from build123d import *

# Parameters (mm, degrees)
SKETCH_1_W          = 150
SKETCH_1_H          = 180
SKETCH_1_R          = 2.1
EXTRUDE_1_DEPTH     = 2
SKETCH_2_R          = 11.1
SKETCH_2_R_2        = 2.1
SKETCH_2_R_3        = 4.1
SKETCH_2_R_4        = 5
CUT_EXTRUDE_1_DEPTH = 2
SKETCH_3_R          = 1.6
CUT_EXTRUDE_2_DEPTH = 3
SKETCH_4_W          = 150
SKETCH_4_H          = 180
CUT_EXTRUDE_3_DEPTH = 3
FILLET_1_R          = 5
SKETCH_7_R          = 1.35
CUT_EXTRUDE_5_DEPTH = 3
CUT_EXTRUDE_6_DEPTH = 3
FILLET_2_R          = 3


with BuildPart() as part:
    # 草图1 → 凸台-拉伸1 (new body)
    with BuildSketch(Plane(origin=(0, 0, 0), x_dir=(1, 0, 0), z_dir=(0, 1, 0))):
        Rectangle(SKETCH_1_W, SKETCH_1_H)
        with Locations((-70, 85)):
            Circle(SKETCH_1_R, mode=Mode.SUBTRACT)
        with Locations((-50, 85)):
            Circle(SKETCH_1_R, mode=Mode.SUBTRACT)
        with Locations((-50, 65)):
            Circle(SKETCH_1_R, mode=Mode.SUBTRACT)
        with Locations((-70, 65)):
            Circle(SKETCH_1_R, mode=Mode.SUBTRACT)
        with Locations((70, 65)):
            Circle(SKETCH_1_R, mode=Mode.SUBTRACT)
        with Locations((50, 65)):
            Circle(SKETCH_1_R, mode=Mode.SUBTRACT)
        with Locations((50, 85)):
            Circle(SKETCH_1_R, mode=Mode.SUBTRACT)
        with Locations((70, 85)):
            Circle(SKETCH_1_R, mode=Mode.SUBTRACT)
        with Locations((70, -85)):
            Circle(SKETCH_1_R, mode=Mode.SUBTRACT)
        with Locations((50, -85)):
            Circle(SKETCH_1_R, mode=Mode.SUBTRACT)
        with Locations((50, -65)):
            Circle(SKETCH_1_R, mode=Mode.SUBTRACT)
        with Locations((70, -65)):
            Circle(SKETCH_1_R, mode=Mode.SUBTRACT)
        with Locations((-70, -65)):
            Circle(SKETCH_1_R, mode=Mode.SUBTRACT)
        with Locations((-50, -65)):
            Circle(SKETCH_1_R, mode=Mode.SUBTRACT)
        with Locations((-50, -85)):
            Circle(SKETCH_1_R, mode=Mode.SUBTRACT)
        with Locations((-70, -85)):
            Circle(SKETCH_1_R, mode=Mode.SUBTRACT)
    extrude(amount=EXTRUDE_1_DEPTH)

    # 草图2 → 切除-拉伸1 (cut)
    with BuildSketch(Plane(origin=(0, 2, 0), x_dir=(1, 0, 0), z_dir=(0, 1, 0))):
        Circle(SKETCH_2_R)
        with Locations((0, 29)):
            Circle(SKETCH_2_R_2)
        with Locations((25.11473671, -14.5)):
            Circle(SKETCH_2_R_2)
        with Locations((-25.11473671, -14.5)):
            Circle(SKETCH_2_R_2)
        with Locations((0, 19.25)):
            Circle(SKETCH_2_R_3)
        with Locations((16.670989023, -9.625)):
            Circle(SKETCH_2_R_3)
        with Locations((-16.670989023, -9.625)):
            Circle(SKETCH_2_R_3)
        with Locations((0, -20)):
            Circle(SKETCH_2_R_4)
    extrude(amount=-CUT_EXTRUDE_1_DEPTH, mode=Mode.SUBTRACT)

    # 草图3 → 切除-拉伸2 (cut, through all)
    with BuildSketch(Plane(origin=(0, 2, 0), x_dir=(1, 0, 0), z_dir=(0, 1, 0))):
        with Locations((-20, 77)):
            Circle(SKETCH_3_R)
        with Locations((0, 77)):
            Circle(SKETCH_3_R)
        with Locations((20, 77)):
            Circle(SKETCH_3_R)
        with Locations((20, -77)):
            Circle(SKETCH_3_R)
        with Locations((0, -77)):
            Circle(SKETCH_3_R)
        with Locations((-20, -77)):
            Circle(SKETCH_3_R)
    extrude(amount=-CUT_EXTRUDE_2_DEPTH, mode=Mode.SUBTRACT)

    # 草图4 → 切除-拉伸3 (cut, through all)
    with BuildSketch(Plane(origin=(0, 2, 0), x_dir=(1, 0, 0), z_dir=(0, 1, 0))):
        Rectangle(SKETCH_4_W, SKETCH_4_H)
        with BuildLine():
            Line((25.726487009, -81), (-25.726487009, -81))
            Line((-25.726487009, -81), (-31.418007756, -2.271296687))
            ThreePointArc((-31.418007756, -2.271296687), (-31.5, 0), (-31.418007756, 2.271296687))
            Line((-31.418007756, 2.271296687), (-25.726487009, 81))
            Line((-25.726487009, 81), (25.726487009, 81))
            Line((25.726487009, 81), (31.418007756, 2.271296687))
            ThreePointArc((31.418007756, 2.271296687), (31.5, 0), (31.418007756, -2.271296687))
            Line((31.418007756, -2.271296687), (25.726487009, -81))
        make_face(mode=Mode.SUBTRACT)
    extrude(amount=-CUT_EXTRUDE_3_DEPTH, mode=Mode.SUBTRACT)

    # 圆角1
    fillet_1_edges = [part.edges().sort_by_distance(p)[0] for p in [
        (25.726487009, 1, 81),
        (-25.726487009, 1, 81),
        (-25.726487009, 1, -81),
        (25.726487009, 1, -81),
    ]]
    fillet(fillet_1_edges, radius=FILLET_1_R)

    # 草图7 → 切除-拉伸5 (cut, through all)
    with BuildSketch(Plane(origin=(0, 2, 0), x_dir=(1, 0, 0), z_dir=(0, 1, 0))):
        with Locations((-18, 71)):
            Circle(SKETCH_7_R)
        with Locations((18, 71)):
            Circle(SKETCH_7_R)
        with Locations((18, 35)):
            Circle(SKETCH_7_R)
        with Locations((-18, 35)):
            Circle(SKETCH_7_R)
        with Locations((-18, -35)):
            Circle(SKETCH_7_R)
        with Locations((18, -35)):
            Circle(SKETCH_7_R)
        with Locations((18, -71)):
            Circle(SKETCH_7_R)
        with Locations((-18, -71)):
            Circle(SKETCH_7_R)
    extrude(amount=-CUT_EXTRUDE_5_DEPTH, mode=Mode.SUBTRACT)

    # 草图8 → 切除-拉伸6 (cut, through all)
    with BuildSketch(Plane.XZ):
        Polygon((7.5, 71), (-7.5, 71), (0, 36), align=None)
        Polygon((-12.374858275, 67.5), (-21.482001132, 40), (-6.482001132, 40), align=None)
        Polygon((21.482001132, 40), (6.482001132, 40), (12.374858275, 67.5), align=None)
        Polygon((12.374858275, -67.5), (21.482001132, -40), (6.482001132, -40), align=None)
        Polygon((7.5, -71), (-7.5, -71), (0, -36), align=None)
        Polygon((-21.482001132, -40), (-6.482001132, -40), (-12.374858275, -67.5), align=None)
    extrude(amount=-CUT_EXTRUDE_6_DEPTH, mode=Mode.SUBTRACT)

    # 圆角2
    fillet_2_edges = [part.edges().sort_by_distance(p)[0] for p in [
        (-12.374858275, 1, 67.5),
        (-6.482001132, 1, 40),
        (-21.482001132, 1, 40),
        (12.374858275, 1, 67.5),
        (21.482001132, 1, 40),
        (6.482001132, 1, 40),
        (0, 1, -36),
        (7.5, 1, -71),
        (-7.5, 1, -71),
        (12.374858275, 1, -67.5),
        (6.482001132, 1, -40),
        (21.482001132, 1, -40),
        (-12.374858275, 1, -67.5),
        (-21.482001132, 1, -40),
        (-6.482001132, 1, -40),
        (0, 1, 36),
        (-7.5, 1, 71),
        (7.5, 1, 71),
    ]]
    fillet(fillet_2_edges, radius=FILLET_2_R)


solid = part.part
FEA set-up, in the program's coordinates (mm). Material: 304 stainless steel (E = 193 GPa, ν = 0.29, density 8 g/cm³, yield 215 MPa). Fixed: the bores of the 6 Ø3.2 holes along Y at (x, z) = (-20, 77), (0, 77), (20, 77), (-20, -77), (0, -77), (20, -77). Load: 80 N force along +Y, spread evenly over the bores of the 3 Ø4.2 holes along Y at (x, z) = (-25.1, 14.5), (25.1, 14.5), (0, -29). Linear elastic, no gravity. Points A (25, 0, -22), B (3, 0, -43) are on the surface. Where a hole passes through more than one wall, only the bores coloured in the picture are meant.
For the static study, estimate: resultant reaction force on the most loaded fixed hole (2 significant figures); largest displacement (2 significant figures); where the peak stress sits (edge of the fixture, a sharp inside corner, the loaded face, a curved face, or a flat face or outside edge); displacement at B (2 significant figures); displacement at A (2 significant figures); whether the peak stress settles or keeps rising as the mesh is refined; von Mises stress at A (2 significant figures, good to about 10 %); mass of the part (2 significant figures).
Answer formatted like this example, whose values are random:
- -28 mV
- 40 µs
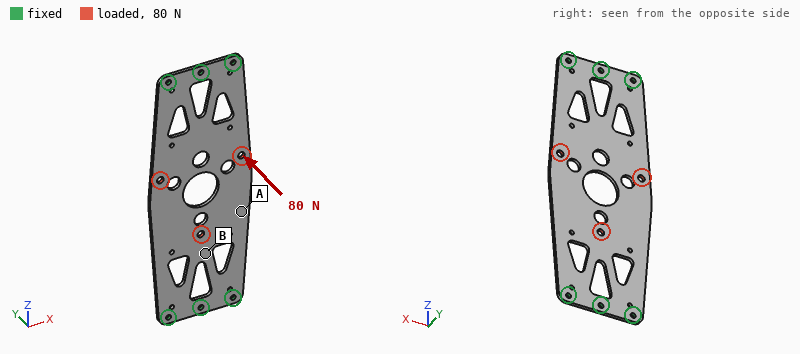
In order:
- 20 N
- 0.26 mm
- edge of the fixture
- 0.11 mm
- 0.19 mm
- keeps rising
- 18 MPa
- 120 g
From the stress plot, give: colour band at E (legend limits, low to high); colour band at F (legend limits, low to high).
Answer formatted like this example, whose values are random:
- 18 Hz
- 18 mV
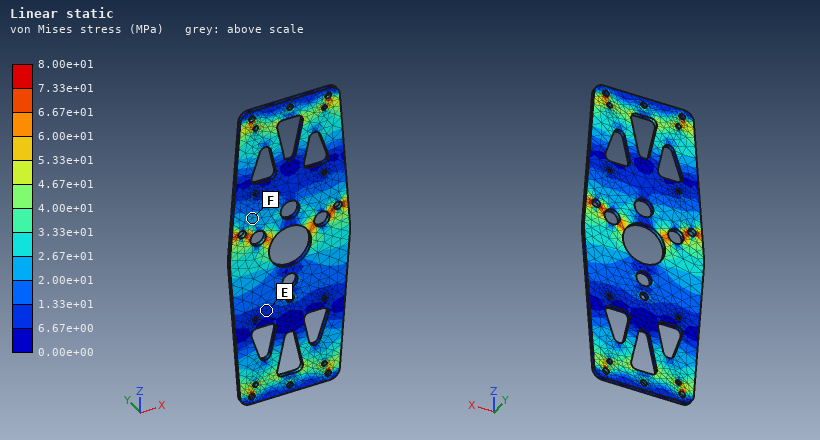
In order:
- 6.67e+00 to 1.33e+01 MPa
- 2.00e+01 to 2.67e+01 MPa
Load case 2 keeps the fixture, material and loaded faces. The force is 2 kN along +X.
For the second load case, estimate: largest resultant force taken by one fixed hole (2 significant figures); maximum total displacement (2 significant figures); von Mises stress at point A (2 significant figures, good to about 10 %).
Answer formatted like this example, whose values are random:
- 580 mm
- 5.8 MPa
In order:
- 730 N
- 33 µm
- 17 MPa
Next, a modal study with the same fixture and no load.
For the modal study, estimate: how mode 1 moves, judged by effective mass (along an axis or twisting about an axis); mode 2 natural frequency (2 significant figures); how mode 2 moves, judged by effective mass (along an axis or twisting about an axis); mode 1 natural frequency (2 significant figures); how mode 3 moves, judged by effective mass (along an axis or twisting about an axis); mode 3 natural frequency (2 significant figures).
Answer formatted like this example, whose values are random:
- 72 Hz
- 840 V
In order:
- along Y
- 700 Hz
- twisting about Z
- 390 Hz
- twisting about X
- 1100 Hz
